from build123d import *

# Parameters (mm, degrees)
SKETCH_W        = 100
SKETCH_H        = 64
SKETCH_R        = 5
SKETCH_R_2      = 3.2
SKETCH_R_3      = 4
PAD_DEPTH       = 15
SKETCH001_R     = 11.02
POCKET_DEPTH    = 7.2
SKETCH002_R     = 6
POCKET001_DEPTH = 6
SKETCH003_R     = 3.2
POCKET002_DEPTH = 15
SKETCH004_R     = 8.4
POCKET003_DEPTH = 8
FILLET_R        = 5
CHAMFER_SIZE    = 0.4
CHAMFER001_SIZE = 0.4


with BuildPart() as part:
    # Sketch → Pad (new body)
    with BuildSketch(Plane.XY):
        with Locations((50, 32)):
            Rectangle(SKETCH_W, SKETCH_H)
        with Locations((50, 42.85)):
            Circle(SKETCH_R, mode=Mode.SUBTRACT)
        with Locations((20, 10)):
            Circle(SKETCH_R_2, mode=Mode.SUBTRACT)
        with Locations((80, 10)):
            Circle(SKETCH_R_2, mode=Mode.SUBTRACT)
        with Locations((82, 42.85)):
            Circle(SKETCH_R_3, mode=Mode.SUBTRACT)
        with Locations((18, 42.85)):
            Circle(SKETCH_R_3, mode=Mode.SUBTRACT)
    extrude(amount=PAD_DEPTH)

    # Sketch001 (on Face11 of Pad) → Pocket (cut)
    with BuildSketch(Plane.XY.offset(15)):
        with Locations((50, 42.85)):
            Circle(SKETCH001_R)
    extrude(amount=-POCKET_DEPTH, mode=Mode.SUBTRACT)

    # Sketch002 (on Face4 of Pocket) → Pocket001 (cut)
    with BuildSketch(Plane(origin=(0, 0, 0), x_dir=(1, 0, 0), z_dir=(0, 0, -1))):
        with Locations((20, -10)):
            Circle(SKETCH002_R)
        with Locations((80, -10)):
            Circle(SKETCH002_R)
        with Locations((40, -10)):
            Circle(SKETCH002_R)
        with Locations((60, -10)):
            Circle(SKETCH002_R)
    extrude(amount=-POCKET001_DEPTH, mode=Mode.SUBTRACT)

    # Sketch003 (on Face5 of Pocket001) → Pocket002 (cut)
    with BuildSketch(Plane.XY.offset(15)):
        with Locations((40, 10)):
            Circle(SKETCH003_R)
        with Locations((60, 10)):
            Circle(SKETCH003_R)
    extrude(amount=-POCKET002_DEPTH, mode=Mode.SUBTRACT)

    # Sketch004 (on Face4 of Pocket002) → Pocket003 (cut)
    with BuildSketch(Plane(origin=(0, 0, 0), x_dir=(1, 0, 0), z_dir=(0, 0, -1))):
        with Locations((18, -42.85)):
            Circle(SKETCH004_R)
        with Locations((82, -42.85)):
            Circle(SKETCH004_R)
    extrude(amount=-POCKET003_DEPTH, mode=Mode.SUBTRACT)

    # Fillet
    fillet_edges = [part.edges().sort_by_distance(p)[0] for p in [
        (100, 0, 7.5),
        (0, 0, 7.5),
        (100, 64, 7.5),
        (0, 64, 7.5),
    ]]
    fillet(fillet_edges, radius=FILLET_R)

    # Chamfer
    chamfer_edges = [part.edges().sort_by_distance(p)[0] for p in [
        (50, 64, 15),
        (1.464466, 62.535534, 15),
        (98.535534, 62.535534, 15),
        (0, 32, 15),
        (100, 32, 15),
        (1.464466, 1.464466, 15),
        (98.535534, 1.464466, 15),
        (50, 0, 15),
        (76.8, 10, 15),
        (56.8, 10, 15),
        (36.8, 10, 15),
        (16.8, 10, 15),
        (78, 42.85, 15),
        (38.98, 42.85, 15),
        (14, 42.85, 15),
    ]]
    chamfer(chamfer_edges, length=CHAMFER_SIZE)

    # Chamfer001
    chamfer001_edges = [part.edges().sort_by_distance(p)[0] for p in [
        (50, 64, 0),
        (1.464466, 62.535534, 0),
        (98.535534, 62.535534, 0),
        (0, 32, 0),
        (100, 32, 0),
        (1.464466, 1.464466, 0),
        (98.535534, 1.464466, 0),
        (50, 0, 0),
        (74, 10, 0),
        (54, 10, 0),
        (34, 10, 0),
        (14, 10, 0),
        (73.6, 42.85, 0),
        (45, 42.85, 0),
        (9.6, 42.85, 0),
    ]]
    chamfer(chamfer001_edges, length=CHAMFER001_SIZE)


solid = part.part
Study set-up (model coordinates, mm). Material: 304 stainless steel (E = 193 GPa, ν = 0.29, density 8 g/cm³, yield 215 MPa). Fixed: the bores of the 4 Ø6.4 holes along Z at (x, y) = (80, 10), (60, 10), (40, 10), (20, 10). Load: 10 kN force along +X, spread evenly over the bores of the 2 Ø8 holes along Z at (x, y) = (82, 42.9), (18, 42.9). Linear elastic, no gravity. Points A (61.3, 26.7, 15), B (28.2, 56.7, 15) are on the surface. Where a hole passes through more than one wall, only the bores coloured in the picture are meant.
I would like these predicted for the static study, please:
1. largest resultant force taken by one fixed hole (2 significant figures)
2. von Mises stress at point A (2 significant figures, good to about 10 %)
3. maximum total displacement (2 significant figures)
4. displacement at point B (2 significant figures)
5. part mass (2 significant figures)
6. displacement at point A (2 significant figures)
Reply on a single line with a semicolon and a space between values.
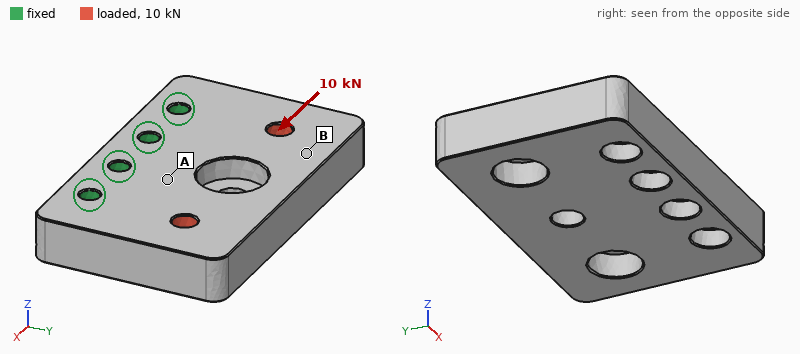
5.3 kN; 22 MPa; 16 µm; 11 µm; 670 g; 3.3 µm
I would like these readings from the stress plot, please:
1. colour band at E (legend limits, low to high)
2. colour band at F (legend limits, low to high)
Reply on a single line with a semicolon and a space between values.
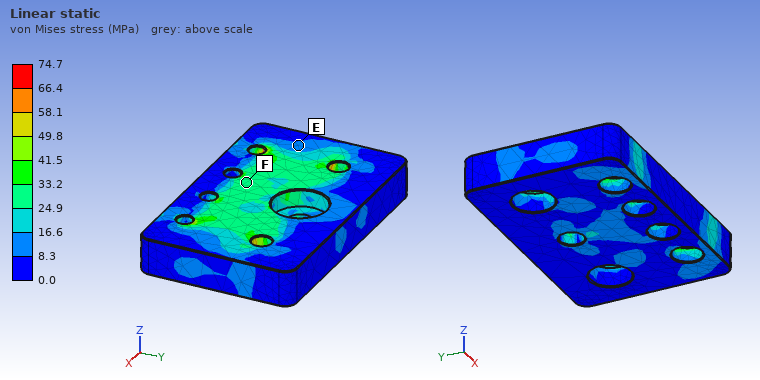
8.3 to 16.6 MPa; 24.9 to 33.2 MPa
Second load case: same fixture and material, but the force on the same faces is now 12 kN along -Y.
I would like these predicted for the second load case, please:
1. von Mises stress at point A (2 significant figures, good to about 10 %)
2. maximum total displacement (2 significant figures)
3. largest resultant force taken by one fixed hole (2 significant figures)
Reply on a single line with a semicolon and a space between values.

17 MPa; 12 µm; 4.1 kN
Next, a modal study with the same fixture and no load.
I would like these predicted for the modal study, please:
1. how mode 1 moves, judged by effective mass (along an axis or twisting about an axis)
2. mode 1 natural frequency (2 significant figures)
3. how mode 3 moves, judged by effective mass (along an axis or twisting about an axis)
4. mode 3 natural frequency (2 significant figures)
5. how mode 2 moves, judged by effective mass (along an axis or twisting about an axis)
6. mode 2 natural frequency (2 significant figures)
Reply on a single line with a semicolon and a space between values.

along Z; 2800 Hz; along X; 8300 Hz; twisting about Y; 4400 Hz
